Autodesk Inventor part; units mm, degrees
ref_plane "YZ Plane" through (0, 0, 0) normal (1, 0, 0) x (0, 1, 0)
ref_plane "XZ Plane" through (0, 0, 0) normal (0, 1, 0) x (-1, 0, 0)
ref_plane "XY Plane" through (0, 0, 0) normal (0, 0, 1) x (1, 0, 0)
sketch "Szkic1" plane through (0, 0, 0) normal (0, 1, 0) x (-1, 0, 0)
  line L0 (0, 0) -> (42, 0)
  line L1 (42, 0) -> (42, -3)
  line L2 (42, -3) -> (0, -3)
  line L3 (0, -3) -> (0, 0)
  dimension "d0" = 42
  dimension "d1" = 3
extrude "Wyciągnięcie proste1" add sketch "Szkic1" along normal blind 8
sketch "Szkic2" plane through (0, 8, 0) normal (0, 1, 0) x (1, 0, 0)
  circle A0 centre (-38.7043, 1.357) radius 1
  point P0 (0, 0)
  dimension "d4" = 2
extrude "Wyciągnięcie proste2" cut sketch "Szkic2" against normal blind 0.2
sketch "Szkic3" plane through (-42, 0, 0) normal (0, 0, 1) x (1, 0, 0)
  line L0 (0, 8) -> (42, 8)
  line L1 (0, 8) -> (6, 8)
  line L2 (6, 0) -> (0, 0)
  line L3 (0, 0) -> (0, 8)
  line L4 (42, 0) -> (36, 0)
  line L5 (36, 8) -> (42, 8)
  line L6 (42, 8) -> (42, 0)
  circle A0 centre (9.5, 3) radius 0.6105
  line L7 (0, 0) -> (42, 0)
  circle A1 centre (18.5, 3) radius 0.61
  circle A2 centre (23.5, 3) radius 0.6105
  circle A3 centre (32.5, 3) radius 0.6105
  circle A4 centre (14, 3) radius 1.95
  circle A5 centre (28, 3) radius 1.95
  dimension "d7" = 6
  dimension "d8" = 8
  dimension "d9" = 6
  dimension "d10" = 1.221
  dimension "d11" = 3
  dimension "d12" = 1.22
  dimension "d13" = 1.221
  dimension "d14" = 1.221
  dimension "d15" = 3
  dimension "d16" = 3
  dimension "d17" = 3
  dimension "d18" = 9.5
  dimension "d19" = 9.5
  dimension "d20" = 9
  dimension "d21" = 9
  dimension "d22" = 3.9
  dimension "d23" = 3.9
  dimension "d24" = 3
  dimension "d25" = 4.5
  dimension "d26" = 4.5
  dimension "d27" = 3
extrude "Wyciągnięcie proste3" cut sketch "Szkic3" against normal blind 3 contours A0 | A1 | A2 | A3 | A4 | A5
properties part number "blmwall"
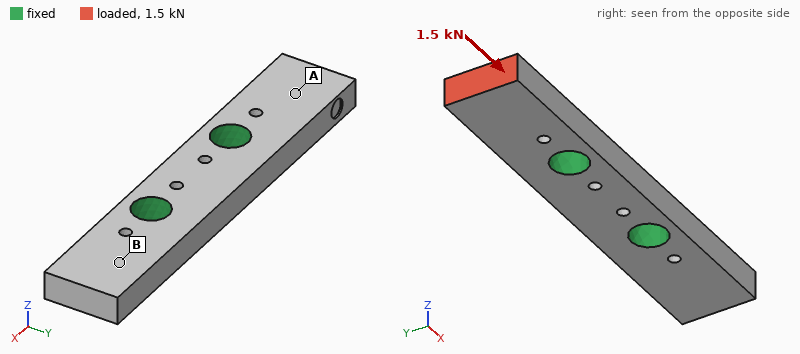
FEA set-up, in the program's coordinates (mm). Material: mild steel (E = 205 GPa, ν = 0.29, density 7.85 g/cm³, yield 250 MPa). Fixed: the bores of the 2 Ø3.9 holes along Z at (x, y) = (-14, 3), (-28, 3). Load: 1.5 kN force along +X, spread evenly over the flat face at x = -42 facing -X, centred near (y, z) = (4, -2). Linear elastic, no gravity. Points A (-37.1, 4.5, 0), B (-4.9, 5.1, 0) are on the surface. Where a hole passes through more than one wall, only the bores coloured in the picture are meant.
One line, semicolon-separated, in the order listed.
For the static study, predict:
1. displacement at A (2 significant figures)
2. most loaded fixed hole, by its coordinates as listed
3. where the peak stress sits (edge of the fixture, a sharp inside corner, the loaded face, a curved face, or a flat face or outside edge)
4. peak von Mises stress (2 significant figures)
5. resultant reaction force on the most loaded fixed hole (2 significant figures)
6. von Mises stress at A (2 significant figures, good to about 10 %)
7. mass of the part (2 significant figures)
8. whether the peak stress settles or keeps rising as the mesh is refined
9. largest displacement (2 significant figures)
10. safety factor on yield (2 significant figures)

3.1 µm; (-28, 3); a curved face; 220 MPa; 1.4 kN; 62 MPa; 7.2 g; settles; 5.4 µm; 1.1
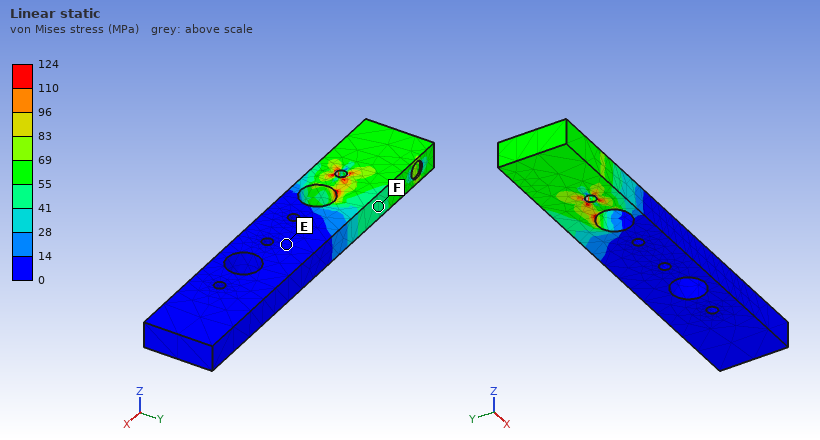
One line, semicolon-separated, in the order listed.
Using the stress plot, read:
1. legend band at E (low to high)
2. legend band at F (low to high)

0 to 14 MPa; 41 to 55 MPa
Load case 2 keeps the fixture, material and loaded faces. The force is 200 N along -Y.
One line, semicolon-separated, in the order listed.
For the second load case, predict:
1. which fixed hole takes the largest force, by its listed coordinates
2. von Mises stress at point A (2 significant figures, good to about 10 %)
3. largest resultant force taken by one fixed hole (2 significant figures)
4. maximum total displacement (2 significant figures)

(-28, 3); 22 MPa; 250 N; 10 µm
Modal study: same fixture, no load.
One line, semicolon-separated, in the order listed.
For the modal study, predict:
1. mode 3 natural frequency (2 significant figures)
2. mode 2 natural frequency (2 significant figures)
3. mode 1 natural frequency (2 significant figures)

27 kHz; 14 kHz; 14 kHz
